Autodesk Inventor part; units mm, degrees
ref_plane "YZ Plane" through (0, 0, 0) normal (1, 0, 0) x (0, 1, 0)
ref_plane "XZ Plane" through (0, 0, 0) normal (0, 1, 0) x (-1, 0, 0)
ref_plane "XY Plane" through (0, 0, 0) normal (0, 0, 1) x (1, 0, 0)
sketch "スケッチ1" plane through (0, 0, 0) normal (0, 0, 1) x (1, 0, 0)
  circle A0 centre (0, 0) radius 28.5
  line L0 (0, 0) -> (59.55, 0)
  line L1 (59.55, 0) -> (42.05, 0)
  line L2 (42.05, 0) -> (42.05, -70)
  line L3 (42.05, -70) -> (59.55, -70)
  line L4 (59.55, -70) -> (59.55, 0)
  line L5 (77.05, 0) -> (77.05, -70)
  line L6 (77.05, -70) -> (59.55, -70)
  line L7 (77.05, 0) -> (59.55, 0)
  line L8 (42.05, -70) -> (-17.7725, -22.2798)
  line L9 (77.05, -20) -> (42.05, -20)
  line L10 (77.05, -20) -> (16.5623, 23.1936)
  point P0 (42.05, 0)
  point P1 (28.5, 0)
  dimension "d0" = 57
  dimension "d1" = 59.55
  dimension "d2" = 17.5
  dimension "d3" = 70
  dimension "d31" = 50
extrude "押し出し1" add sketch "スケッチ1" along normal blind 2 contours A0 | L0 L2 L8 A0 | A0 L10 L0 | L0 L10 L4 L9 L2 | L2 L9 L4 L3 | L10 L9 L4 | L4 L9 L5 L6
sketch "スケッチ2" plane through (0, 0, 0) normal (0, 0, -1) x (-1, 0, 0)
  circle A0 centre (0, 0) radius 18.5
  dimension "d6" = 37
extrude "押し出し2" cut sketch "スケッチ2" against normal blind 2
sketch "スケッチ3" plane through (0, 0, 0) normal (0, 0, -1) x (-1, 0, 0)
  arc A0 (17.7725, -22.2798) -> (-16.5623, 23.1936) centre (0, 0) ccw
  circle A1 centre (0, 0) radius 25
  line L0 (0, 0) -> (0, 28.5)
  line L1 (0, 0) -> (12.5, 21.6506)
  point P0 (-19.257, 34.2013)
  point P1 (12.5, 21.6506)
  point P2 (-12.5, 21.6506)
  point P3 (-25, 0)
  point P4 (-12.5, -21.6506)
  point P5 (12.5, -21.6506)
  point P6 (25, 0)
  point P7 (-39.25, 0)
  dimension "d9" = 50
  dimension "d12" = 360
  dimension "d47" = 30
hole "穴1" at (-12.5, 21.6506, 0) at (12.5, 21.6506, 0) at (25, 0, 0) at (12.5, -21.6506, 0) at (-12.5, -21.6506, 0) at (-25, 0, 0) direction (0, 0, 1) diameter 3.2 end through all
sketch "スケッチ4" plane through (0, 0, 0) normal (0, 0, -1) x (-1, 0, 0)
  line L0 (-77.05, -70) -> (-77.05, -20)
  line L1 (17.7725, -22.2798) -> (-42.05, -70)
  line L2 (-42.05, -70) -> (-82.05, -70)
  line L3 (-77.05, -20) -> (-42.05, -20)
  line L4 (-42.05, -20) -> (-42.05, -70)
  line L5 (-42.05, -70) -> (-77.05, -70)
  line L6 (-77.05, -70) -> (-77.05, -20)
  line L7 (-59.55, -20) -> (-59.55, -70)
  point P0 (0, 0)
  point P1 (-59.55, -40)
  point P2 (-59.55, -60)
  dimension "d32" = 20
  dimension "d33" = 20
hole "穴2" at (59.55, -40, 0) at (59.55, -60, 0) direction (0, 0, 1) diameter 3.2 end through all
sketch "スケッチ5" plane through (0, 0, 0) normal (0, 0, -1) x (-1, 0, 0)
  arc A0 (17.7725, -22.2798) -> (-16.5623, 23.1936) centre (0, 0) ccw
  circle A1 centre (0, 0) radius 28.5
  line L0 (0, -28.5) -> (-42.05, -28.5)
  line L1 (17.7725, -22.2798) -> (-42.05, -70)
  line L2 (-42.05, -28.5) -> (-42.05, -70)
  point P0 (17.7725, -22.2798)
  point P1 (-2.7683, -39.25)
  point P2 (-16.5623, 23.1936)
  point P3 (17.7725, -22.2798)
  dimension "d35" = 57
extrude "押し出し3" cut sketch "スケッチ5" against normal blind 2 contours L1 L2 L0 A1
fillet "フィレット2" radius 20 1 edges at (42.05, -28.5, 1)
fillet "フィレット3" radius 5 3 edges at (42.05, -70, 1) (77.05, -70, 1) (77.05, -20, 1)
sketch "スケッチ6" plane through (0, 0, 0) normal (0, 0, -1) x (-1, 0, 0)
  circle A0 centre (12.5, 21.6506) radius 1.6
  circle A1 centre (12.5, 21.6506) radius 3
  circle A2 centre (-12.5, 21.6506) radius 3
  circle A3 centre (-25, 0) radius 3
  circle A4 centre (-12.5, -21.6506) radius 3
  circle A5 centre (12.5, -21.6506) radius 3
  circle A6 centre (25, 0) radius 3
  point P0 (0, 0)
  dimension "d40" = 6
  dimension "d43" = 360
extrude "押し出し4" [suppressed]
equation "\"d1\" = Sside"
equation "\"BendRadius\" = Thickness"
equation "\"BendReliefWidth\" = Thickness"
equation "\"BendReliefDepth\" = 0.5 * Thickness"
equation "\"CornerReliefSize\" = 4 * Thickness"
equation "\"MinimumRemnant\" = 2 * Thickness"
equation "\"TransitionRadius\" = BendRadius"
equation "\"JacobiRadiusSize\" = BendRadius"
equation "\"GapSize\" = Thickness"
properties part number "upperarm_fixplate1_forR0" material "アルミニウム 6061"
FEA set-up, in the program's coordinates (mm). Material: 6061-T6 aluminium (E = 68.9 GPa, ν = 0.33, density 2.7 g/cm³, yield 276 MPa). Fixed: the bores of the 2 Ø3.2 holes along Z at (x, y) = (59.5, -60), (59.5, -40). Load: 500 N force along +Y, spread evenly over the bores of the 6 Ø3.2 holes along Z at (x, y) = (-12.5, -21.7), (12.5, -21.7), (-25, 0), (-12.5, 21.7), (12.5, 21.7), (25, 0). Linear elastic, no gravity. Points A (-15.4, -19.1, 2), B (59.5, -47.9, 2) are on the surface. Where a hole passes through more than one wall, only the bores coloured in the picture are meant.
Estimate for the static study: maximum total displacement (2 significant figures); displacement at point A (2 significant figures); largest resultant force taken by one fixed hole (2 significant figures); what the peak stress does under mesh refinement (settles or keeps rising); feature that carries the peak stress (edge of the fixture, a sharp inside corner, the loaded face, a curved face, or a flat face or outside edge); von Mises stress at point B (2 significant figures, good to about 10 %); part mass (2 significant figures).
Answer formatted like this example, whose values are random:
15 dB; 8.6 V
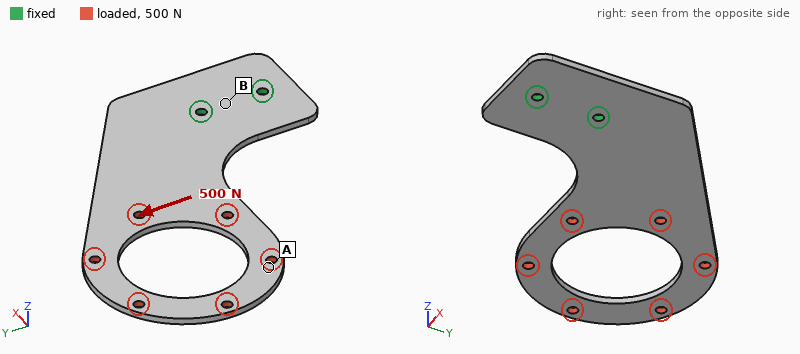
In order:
0.39 mm; 0.31 mm; 1.4 kN; keeps rising; edge of the fixture; 32 MPa; 24 g
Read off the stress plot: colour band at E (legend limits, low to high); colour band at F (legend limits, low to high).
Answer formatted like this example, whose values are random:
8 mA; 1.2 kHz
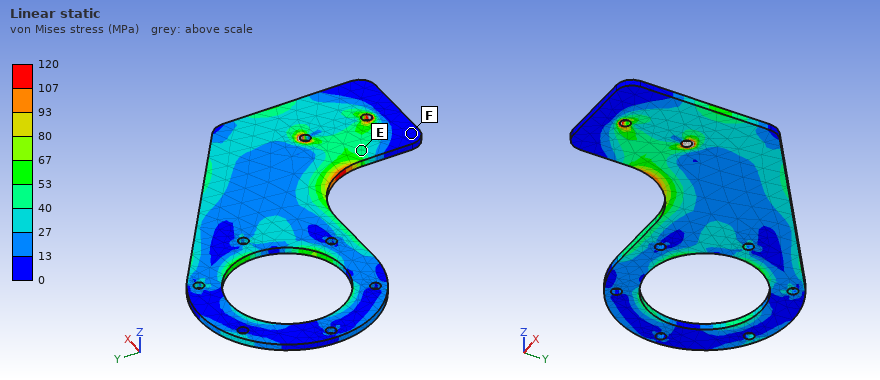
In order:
40 to 53 MPa; 0 to 13 MPa
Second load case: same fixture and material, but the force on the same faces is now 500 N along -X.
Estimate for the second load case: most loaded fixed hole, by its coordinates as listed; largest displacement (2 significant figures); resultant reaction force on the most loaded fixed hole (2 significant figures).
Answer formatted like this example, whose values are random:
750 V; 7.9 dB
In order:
(59.5, -40); 0.22 mm; 1.4 kN
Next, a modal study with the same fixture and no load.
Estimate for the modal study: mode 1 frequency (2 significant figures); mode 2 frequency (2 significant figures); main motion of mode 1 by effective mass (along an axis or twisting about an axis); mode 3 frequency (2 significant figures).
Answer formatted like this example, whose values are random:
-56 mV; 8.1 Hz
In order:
180 Hz; 550 Hz; along Z; 900 Hz
